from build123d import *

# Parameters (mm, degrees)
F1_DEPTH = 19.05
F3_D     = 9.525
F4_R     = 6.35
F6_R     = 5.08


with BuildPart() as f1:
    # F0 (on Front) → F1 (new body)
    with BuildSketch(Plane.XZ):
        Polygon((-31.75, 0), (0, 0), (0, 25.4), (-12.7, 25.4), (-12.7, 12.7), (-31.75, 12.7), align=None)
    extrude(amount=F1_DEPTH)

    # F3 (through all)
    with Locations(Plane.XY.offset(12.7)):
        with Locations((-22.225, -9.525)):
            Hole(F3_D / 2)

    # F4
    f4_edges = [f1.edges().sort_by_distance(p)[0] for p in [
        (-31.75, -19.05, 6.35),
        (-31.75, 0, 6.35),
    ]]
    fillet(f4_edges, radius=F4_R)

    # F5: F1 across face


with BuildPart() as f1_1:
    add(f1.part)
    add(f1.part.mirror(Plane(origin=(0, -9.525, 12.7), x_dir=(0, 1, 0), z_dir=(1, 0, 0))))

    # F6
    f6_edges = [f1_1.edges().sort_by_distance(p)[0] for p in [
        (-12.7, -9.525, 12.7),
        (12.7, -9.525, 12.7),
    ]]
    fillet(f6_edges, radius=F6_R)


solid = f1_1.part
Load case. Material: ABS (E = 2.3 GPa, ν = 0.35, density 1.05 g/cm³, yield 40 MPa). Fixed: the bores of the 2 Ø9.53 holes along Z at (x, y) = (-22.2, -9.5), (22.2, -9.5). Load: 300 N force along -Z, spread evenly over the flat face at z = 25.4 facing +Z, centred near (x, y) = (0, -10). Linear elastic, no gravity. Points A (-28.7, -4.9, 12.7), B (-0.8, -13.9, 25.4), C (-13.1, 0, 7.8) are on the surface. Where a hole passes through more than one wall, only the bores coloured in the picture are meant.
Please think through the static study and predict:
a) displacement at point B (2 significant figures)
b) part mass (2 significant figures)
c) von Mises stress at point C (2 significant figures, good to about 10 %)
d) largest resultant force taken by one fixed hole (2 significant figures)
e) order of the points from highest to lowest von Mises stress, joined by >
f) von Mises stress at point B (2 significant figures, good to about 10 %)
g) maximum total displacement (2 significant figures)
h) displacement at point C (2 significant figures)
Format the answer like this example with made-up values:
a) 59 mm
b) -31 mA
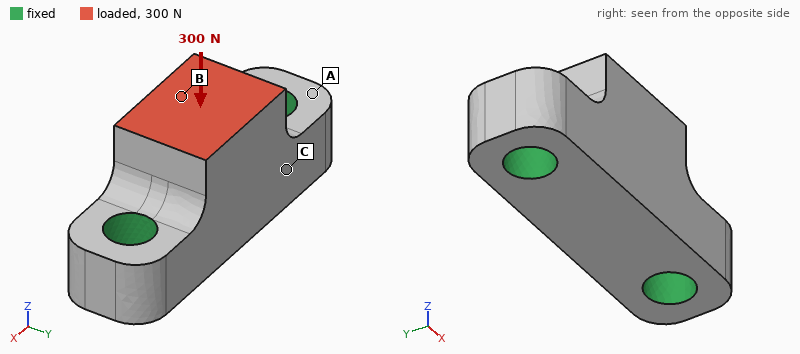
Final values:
a) 13 µm
b) 20 g
c) 0.97 MPa
d) 160 N
e) C > B > A
f) 0.52 MPa
g) 13 µm
h) 6.4 µm
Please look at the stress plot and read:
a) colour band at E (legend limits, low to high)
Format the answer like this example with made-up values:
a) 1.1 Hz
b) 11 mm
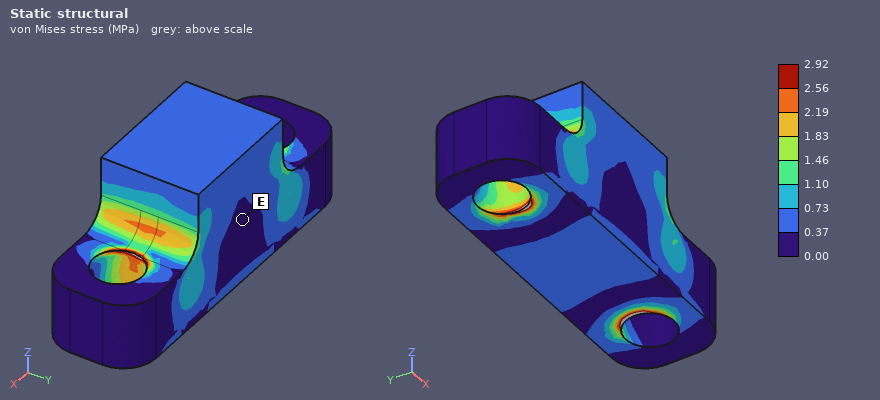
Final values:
a) 0.00 to 0.37 MPa
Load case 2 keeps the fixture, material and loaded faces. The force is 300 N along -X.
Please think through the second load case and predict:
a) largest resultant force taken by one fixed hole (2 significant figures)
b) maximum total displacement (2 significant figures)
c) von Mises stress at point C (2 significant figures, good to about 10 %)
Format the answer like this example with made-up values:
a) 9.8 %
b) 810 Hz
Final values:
a) 210 N
b) 28 µm
c) 0.70 MPa
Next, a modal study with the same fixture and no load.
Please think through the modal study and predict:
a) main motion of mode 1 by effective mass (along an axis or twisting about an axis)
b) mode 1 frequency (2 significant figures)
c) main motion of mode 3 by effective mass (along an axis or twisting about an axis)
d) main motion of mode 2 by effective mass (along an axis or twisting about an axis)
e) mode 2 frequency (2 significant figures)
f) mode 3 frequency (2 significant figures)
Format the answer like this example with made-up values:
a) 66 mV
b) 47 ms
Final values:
a) along Y
b) 4400 Hz
c) along Y
d) along Z
e) 7500 Hz
f) 8800 Hz
